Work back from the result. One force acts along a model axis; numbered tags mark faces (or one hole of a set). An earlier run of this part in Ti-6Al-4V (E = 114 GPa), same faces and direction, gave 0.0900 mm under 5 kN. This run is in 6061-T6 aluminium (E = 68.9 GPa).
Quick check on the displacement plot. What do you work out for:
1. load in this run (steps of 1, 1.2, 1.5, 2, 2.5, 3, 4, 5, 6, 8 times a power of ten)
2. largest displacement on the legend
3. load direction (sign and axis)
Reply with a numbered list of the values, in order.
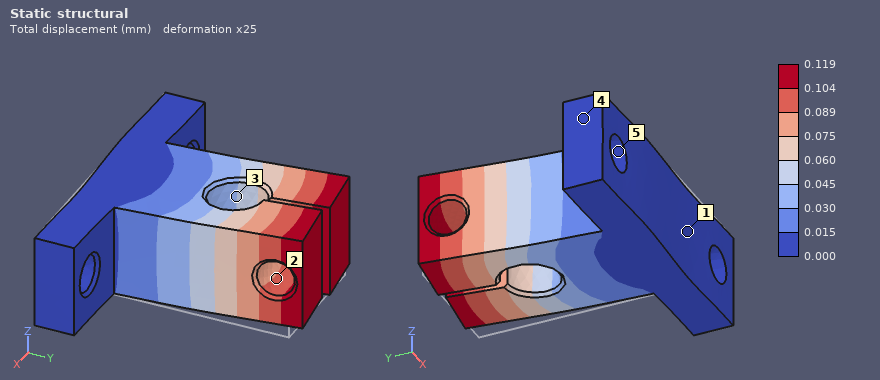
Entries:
1. 4 kN
2. 0.119 mm
3. -X
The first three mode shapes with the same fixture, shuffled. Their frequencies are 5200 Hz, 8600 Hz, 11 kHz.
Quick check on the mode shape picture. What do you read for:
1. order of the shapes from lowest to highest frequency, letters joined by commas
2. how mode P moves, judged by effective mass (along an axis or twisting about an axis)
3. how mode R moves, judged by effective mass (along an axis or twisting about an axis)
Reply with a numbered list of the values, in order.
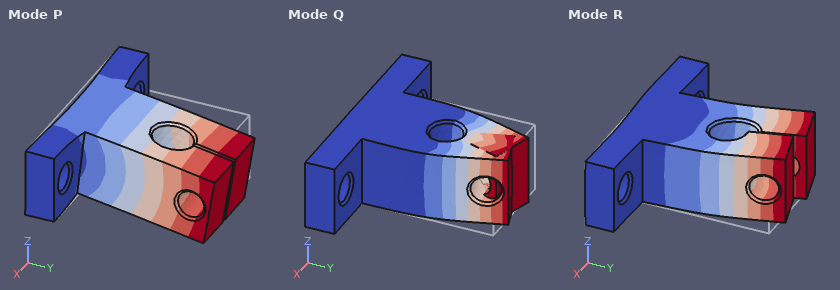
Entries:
1. P, R, Q
2. along Z
3. along X
